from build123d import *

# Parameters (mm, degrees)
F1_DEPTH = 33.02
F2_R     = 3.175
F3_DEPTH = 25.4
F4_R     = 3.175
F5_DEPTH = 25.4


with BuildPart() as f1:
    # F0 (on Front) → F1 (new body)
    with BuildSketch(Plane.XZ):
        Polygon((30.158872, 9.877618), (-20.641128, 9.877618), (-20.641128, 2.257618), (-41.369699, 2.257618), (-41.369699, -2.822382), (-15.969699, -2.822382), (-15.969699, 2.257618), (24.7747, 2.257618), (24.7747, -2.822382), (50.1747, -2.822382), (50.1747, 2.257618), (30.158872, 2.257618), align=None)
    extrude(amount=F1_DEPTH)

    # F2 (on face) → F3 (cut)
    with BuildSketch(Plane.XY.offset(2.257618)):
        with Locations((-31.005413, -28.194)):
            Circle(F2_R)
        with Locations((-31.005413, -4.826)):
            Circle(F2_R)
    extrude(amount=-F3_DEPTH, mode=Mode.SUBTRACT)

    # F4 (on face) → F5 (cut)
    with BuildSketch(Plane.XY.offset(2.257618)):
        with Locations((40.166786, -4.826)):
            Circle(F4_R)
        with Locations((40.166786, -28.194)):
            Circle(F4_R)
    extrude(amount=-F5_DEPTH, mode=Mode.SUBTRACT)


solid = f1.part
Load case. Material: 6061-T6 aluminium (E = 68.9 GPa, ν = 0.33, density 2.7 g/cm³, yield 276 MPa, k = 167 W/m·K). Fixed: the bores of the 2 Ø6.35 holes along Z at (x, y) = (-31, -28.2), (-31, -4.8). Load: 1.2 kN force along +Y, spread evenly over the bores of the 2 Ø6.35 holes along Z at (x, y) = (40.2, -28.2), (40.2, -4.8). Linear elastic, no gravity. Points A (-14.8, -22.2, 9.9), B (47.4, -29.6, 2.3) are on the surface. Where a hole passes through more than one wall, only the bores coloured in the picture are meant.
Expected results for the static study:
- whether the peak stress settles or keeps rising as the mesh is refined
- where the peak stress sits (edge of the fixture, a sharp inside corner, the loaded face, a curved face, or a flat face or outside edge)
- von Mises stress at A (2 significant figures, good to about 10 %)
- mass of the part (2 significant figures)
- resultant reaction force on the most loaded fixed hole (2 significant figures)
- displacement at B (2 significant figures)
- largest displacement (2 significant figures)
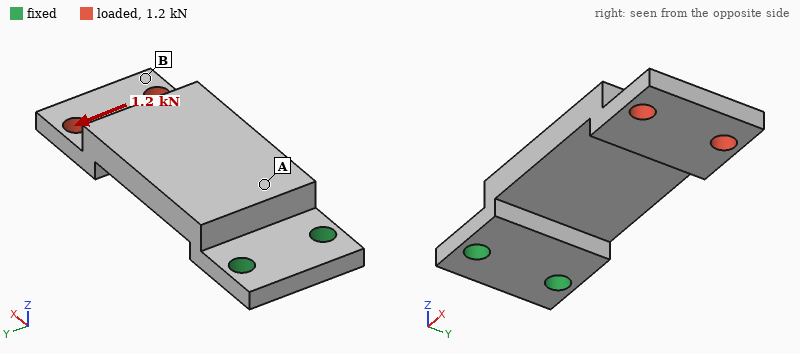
keeps rising
a sharp inside corner
69 MPa
56 g
3.4 kN
0.31 mm
0.36 mm
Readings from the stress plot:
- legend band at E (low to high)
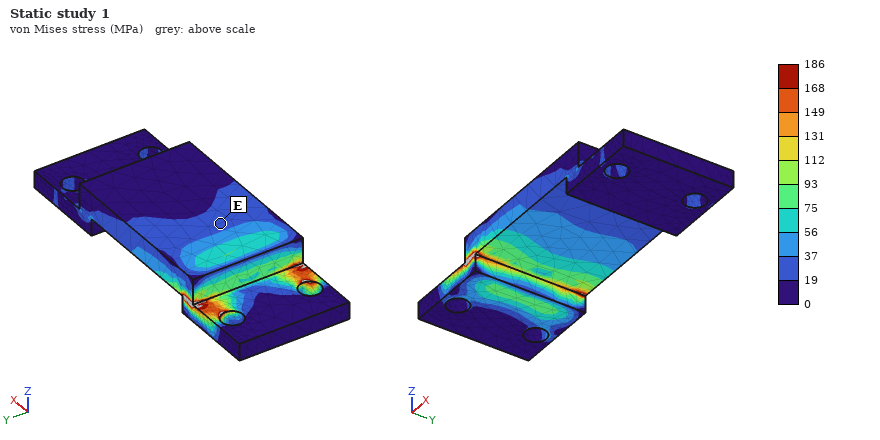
19 to 37 MPa
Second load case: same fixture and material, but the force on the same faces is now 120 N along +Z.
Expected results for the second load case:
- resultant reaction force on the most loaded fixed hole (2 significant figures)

61 N
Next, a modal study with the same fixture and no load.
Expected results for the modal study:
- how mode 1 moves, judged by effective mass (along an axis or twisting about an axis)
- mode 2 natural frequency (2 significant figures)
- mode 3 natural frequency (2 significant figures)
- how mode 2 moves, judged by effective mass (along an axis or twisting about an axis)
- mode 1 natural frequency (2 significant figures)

along Z
2500 Hz
4600 Hz
along Y
690 Hz
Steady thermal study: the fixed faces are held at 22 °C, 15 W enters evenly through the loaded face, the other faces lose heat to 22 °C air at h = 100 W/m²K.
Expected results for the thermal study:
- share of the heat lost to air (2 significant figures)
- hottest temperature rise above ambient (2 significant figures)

50 %
22 K
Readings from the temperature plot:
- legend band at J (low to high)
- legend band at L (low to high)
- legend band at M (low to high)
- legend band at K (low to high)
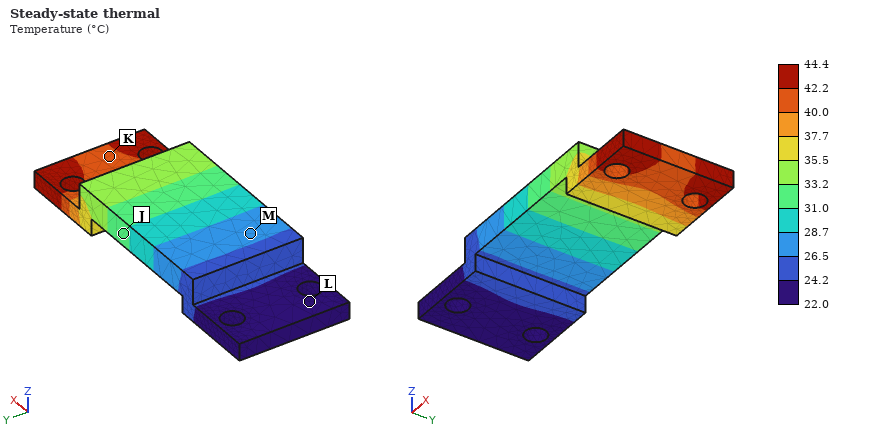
31.0 to 33.2 °C
22.0 to 24.2 °C
26.5 to 28.7 °C
40.0 to 42.2 °C
